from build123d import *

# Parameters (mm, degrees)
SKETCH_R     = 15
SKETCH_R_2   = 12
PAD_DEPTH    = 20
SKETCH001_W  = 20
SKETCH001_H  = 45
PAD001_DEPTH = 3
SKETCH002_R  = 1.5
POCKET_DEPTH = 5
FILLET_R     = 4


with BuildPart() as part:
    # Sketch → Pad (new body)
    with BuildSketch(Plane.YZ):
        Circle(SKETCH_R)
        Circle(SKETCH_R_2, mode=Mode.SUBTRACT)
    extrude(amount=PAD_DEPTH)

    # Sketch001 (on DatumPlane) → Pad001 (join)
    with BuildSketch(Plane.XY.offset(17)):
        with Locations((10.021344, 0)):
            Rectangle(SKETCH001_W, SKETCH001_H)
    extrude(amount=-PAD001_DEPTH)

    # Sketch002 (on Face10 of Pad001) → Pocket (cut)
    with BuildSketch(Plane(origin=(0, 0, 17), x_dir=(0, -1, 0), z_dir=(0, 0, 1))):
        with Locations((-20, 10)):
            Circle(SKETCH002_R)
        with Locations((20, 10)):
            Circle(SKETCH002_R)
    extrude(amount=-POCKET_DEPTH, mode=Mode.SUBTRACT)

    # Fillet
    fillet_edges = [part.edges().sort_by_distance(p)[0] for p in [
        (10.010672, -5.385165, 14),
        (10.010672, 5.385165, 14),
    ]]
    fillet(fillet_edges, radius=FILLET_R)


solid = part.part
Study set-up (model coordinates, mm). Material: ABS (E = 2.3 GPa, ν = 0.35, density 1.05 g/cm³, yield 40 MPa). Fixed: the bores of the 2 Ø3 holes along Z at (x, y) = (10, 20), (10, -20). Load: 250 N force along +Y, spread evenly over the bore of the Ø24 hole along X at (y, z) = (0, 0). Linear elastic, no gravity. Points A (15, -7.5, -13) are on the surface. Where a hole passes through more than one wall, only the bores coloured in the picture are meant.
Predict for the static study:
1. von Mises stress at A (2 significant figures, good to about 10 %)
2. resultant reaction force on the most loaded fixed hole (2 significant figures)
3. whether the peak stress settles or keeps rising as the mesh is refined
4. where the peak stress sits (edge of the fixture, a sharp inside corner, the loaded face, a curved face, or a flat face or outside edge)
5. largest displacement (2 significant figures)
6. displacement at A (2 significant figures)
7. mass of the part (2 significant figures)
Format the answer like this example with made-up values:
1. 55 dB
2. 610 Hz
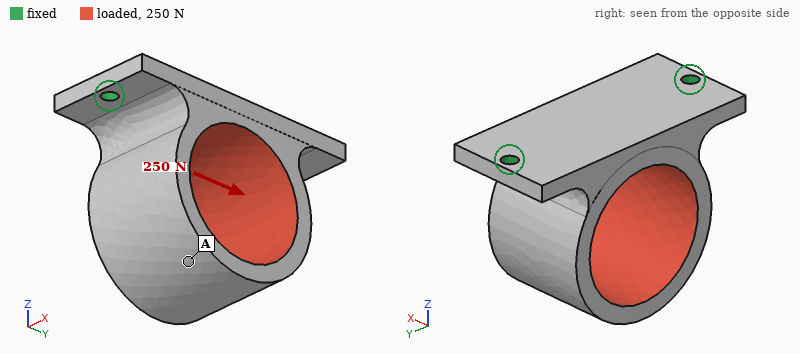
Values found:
1. 6.9 MPa
2. 170 N
3. keeps rising
4. edge of the fixture
5. 0.68 mm
6. 0.67 mm
7. 8.7 g
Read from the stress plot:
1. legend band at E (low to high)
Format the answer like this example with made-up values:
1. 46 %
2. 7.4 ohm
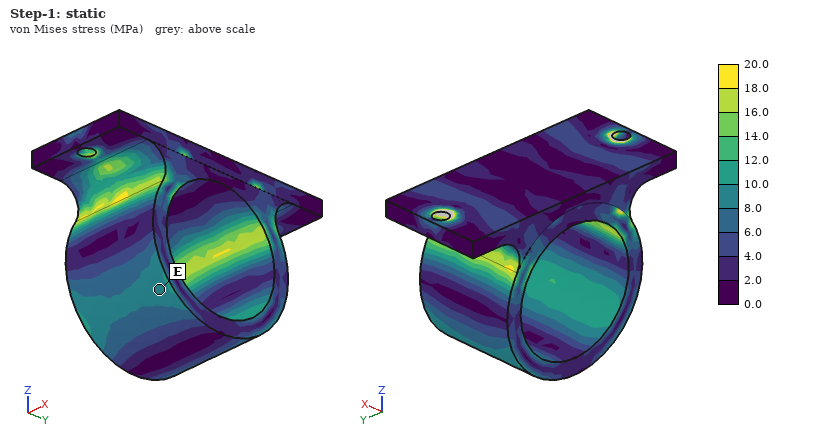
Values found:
1. 8.0 to 10.0 MPa
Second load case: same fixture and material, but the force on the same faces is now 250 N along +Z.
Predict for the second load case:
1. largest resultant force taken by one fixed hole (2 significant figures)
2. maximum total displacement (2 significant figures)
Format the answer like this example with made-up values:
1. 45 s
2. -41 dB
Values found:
1. 150 N
2. 0.16 mm
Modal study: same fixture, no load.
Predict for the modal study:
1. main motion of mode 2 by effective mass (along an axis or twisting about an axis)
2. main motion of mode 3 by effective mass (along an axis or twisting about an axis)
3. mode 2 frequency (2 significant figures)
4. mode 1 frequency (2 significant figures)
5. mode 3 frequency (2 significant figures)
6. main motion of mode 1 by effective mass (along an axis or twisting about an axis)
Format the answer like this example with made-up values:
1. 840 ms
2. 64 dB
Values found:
1. along Y
2. along Z
3. 1400 Hz
4. 710 Hz
5. 2400 Hz
6. along X
